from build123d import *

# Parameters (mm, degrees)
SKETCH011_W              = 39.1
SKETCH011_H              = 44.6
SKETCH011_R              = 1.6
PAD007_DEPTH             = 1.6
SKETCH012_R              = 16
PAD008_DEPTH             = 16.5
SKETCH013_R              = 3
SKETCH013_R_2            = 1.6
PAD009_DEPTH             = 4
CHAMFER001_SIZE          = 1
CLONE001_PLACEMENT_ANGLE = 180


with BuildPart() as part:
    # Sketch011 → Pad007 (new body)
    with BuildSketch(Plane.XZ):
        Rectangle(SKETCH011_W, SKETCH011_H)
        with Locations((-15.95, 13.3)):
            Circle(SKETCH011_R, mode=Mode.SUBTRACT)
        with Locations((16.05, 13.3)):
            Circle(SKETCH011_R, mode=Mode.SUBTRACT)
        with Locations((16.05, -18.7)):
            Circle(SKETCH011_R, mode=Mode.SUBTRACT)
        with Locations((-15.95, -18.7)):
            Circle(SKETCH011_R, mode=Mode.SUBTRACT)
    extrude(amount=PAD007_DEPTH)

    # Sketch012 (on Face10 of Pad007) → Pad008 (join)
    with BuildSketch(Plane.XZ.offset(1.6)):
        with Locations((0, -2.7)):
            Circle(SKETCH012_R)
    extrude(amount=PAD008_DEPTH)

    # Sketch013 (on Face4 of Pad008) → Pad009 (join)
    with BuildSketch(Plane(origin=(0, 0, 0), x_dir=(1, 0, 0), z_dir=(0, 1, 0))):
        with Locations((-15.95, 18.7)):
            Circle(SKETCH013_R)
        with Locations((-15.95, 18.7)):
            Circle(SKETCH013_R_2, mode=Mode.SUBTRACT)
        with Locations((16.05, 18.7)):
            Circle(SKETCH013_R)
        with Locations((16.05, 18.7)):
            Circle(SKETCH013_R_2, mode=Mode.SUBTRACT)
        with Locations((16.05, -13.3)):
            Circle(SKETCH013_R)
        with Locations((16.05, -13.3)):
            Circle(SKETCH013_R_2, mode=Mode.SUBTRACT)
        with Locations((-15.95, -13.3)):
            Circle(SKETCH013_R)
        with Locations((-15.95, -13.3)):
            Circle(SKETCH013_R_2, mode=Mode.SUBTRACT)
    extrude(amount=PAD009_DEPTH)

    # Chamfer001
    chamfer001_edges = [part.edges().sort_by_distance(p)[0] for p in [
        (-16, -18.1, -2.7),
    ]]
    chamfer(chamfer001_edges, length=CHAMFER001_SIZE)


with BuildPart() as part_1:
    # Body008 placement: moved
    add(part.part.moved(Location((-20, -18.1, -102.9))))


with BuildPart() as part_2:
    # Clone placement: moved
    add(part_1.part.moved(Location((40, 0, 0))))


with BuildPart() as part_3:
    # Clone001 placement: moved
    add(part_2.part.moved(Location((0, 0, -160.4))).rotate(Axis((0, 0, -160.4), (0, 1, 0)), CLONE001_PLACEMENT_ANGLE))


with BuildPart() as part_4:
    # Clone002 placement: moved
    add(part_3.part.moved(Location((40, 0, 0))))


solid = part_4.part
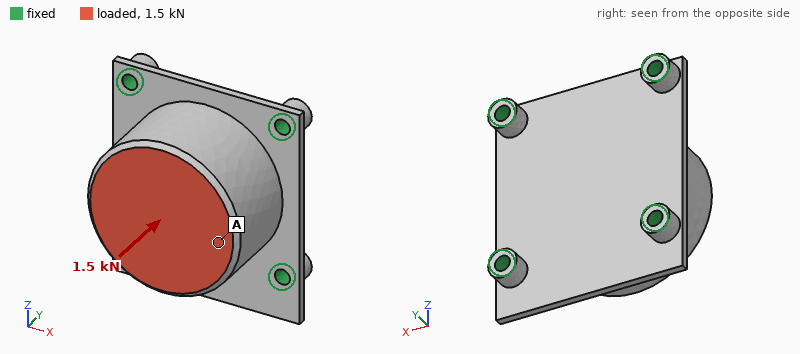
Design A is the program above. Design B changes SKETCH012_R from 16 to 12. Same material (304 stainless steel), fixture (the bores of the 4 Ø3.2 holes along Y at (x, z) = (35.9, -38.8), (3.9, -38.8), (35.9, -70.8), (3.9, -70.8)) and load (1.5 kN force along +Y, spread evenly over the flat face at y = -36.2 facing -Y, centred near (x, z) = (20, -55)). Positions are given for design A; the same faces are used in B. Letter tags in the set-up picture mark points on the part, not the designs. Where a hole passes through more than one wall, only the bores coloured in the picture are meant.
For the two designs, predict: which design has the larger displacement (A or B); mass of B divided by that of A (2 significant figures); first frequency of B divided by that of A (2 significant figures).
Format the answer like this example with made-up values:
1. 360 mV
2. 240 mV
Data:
1. B
2. 0.64
3. 0.72
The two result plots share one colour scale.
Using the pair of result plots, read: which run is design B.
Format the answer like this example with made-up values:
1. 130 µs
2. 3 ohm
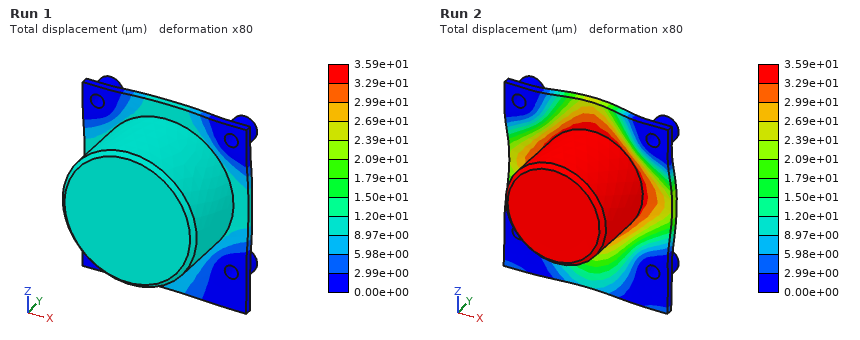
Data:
1. Run 2
